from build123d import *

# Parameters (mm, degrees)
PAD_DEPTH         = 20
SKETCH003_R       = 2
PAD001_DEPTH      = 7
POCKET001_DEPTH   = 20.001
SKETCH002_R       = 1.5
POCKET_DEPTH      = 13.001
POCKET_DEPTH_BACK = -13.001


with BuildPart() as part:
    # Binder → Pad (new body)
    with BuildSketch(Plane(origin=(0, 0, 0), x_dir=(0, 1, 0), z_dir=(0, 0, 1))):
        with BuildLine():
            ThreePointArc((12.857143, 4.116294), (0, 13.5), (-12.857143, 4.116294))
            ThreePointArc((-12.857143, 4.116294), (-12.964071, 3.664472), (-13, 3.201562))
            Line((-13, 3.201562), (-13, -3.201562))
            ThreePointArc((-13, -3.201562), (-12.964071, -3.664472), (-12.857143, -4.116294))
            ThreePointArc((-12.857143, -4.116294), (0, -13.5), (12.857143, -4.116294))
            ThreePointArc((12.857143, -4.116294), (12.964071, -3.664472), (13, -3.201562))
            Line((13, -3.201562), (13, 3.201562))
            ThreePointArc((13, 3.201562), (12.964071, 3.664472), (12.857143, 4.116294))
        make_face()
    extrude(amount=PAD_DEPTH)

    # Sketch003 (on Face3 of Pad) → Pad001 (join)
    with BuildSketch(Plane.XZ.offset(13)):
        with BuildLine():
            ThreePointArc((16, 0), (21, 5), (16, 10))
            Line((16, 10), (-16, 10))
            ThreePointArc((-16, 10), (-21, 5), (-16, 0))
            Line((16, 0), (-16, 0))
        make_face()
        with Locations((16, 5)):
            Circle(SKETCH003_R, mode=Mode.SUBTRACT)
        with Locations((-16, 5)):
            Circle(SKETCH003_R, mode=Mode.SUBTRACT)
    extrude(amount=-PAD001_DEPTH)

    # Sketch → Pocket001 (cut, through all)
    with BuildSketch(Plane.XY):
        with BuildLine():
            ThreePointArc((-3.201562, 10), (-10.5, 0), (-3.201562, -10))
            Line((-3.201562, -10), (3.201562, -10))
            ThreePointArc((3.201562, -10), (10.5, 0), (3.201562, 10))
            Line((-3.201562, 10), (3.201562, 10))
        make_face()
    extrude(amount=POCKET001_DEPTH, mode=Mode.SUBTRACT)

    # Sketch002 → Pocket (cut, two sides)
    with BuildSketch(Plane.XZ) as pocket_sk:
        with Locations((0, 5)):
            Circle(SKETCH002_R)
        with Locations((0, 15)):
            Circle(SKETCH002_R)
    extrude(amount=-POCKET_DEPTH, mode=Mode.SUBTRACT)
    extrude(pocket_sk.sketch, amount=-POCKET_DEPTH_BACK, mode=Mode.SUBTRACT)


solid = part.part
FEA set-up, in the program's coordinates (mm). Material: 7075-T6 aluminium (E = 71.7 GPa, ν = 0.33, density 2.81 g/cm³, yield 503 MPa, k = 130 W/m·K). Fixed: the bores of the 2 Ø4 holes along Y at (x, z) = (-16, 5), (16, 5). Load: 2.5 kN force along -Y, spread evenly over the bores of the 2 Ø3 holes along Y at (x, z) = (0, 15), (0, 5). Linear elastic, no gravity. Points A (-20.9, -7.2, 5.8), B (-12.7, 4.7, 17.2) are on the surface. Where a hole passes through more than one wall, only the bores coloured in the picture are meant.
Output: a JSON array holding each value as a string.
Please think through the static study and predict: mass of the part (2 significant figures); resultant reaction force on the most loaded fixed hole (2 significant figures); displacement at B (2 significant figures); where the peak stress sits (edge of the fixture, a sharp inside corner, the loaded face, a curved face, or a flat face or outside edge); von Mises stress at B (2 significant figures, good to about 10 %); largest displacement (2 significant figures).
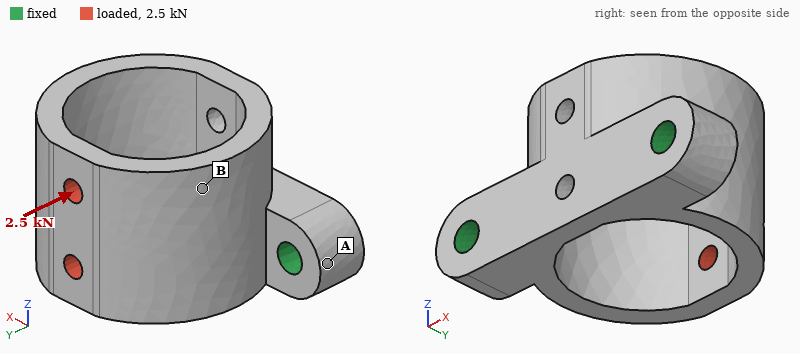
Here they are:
["16 g", "1.4 kN", "0.066 mm", "the loaded face", "83 MPa", "0.13 mm"]
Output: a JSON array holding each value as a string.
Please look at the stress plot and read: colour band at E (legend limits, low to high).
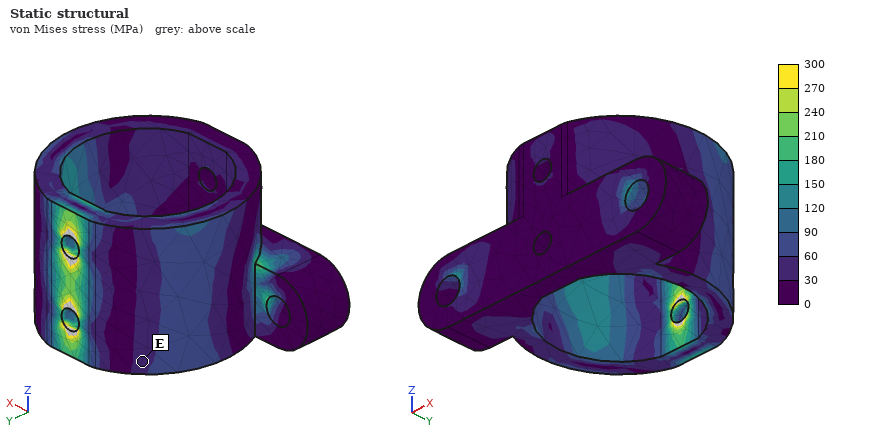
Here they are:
["30 to 60 MPa"]
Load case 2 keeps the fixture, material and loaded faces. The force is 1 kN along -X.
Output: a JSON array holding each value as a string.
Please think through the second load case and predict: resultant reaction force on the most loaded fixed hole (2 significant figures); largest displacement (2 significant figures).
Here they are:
["810 N", "90 µm"]
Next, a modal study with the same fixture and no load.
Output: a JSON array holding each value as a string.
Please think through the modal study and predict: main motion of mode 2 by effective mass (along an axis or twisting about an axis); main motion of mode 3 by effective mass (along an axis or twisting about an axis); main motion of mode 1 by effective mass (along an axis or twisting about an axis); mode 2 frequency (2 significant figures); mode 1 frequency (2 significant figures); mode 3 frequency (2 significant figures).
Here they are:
["along X", "twisting about Y", "along Z", "7700 Hz", "6700 Hz", "14 kHz"]
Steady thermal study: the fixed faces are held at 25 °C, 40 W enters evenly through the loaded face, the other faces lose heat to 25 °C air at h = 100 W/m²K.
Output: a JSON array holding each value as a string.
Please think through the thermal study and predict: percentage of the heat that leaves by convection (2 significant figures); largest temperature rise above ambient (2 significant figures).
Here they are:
["26 %", "70 K"]
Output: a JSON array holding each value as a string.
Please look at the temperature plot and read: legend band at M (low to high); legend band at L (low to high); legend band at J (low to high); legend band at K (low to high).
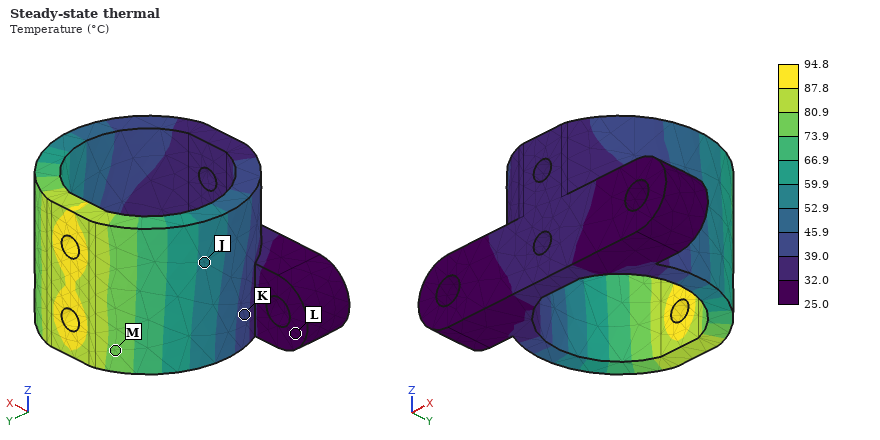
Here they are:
["73.9 to 80.9 °C", "25.0 to 32.0 °C", "52.9 to 59.9 °C", "39.0 to 45.9 °C"]
